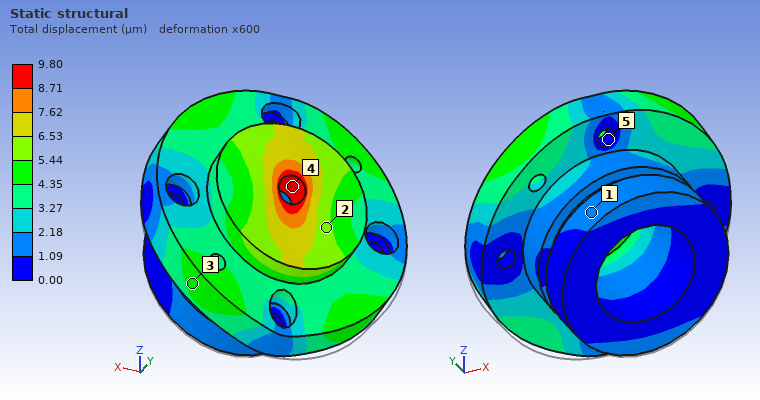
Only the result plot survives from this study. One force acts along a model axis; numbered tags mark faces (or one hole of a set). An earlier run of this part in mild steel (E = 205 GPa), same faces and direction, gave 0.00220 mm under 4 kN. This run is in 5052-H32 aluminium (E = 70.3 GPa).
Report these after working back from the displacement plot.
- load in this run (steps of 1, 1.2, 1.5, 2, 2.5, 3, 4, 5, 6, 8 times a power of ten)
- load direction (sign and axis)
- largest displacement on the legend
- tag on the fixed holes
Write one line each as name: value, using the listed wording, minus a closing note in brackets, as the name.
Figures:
load in this run: 6 kN
load direction: +Z
largest displacement on the legend: 9.80 µm
tag on the fixed holes: 5
